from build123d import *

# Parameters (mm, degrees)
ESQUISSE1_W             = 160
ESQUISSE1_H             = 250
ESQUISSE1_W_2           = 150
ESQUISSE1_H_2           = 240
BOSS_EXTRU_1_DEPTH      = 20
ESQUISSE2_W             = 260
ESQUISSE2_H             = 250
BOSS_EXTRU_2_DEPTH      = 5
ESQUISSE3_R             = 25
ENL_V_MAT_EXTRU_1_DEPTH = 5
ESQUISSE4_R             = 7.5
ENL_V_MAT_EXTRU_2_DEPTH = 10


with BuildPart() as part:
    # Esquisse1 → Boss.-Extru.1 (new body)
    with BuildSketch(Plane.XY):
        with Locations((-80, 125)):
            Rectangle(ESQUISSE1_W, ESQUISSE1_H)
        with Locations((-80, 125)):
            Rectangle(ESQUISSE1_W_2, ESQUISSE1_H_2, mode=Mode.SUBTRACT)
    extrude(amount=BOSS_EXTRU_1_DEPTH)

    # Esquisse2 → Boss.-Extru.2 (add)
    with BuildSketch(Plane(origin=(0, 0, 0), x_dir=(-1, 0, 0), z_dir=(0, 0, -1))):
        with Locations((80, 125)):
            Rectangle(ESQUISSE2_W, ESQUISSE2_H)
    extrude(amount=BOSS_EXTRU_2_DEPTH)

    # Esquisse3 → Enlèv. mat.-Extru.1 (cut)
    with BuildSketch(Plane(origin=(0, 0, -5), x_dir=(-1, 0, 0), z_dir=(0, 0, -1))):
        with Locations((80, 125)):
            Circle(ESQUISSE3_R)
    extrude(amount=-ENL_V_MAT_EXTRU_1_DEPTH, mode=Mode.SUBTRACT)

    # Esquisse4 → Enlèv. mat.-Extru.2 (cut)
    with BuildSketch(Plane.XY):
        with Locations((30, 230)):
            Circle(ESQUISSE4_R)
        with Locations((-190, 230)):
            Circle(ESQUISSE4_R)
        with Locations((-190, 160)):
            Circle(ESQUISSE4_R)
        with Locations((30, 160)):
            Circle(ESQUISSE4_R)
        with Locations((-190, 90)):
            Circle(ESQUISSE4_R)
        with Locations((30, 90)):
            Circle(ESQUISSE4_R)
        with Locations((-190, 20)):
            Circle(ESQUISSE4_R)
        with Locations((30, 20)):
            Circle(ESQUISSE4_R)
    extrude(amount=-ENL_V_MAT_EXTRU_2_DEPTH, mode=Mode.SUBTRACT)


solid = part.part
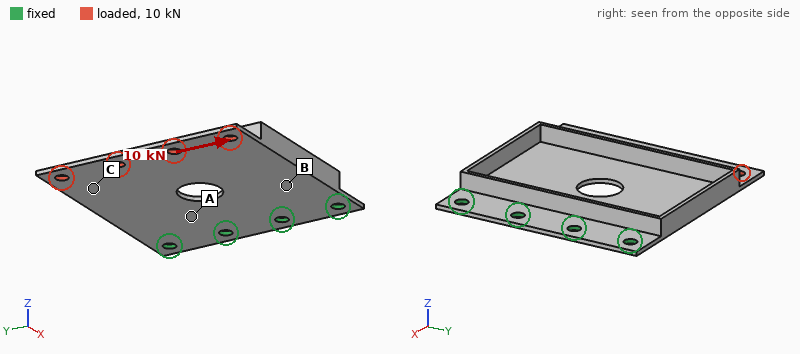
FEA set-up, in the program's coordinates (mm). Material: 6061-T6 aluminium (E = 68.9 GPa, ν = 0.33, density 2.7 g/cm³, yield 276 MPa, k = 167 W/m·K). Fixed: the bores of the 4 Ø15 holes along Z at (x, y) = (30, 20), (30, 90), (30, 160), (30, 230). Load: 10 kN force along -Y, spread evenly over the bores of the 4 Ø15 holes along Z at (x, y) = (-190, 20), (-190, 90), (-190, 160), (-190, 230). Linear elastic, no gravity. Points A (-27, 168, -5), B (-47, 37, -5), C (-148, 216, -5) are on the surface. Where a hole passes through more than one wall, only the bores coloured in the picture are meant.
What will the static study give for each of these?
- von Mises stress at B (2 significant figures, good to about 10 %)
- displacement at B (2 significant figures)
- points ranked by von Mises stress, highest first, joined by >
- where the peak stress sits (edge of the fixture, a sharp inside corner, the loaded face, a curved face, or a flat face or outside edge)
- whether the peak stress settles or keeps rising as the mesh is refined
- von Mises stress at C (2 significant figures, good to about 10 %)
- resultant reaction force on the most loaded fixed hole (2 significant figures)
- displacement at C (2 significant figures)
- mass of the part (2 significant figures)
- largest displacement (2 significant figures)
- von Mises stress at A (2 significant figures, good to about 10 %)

26 MPa
0.062 mm
B > A > C
edge of the fixture
keeps rising
7.4 MPa
9.7 kN
0.15 mm
1.0 kg
0.23 mm
15 MPa
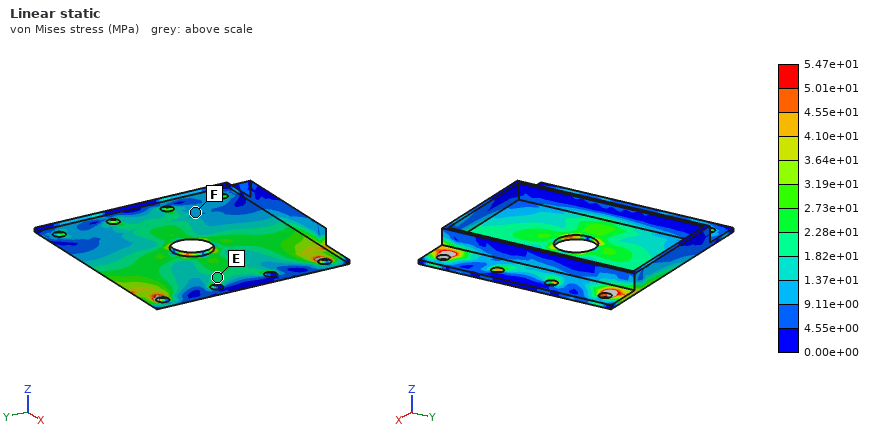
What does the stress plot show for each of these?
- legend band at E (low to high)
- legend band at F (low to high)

1.82e+01 to 2.28e+01 MPa
9.11e+00 to 1.37e+01 MPa
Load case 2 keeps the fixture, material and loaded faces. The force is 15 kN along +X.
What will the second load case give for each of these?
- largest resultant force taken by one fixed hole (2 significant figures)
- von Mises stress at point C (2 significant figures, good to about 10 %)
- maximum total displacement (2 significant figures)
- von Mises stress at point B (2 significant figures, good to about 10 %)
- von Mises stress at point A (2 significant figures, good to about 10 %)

4.1 kN
14 MPa
0.20 mm
15 MPa
14 MPa
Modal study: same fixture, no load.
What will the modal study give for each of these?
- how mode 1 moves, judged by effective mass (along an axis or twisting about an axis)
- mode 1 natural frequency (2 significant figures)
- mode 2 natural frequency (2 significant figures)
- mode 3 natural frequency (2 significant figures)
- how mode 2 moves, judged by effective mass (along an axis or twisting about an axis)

along Z
88 Hz
180 Hz
690 Hz
twisting about X
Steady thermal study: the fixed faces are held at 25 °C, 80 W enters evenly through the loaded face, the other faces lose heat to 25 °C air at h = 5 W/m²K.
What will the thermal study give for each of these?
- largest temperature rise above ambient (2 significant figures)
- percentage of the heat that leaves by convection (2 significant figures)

70 K
31 %
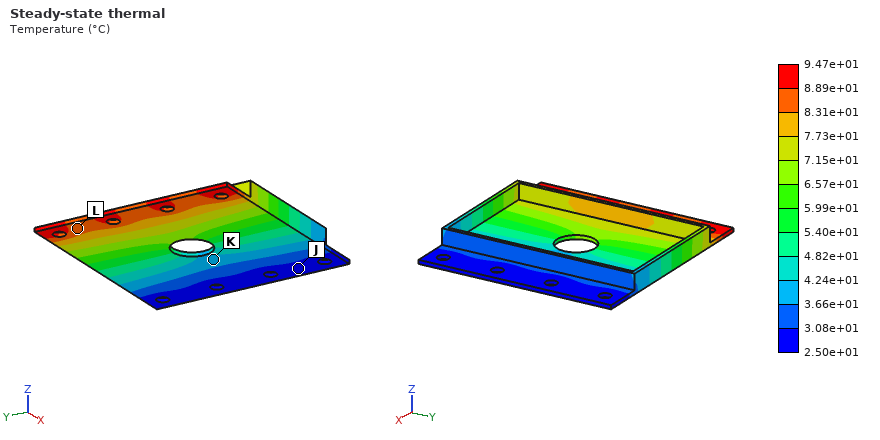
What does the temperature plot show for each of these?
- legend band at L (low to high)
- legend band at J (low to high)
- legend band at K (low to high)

8.31e+01 to 8.89e+01 °C
2.50e+01 to 3.08e+01 °C
3.66e+01 to 4.24e+01 °C
